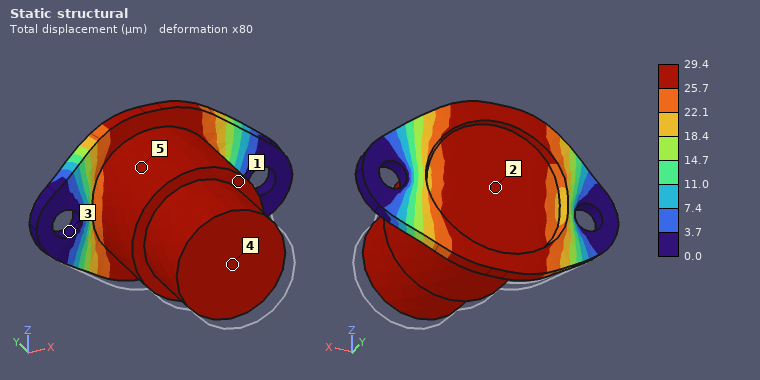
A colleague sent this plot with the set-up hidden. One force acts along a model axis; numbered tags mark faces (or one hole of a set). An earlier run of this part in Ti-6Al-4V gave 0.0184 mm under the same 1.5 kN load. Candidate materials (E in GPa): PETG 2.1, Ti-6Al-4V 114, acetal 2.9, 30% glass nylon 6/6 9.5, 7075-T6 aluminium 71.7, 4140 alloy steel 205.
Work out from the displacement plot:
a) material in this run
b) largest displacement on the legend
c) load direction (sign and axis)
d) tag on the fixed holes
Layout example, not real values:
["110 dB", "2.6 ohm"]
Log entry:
["7075-T6 aluminium", "29.4 µm", "+Y", "3"]
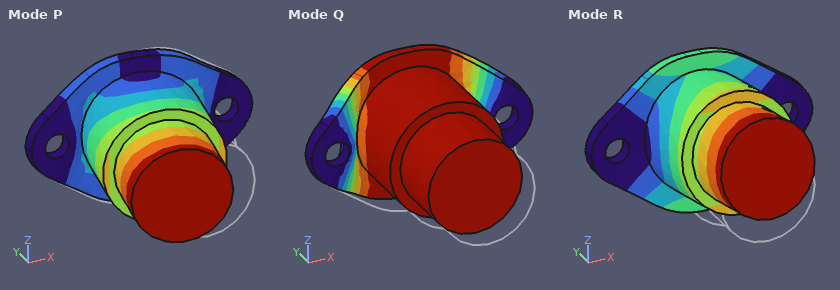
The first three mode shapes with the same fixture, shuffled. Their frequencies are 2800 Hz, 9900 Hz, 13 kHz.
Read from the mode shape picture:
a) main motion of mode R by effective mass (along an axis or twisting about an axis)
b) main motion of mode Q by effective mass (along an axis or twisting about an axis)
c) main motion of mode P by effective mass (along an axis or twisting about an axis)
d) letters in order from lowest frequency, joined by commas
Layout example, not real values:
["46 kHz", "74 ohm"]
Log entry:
["along Z", "along Y", "along X", "R, P, Q"]
